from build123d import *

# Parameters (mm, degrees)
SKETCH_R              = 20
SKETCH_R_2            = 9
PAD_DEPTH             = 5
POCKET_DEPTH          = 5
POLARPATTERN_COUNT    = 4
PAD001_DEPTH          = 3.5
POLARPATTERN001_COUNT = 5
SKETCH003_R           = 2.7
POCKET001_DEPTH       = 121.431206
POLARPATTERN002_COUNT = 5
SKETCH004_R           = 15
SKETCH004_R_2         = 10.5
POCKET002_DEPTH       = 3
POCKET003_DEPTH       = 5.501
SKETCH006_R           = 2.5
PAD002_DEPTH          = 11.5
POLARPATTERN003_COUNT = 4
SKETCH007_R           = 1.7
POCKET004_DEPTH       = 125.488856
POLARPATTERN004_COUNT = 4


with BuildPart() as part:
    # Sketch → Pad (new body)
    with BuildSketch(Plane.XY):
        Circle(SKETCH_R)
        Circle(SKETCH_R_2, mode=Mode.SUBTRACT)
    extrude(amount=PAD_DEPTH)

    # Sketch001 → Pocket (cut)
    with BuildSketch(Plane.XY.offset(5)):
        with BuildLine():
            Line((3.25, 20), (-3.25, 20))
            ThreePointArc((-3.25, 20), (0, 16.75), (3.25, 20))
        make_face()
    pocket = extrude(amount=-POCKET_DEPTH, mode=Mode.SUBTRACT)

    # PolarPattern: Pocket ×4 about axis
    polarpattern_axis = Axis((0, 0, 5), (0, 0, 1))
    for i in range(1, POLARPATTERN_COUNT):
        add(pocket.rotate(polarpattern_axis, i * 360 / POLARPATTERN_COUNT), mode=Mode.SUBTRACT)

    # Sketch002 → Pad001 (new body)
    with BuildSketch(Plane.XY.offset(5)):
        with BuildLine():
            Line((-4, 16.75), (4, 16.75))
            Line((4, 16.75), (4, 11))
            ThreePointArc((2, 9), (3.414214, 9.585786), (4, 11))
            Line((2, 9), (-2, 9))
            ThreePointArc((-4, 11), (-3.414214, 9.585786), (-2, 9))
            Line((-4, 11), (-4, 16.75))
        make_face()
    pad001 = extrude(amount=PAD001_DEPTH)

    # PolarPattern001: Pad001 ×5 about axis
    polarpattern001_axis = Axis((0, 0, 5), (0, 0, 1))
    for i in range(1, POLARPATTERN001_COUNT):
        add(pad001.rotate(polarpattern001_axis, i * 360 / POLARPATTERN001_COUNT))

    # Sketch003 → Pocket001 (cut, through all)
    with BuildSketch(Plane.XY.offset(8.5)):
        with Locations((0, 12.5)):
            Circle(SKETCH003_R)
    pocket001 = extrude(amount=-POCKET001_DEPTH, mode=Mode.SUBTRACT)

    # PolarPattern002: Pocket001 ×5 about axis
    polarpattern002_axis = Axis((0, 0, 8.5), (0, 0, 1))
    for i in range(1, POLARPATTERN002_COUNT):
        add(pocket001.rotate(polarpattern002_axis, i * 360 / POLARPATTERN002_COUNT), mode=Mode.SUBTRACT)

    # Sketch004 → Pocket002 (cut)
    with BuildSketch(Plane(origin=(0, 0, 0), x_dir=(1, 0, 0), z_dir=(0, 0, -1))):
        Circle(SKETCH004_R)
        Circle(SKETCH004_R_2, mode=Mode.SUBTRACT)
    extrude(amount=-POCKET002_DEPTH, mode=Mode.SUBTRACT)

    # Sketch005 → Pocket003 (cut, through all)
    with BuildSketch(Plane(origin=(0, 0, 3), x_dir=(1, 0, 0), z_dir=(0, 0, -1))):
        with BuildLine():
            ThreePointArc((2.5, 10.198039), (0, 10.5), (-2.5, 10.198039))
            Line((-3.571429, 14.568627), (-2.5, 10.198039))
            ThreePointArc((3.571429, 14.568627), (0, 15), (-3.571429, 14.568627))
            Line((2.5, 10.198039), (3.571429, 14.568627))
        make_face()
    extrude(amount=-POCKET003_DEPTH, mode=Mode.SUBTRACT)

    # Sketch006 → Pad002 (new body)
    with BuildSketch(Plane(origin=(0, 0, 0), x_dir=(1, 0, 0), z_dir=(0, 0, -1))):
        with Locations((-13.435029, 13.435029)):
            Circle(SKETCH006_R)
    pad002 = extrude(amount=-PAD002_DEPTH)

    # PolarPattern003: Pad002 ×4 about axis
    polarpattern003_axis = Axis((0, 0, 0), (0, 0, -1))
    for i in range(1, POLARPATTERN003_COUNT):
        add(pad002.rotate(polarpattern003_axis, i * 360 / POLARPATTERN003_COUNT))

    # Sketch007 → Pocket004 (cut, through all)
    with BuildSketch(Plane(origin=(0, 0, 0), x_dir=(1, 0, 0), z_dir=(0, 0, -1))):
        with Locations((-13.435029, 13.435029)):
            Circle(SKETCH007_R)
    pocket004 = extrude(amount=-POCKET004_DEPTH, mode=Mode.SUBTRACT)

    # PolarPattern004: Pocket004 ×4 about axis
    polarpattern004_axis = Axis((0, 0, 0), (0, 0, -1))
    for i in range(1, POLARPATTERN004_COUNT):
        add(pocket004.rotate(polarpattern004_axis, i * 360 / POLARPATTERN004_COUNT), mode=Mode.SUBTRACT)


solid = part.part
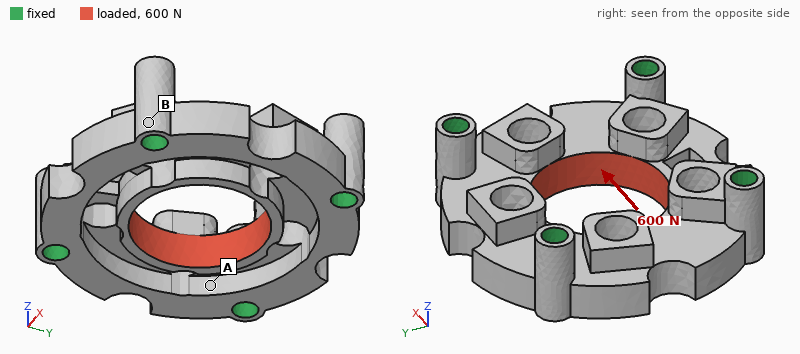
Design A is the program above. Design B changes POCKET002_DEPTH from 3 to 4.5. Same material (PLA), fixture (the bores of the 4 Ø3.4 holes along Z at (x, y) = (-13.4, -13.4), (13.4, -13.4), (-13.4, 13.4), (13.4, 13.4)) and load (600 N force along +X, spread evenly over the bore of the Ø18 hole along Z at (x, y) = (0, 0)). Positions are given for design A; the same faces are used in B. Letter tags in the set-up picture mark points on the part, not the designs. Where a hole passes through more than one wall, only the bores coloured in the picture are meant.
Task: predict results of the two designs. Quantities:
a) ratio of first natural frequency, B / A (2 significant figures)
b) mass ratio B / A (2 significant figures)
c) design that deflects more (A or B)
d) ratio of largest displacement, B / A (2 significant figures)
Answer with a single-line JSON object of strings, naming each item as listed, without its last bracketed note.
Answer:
{"ratio of first natural frequency, B / A": "0.71", "mass ratio B / A": "0.92", "design that deflects more": "B", "ratio of largest displacement, B / A": "2.2"}
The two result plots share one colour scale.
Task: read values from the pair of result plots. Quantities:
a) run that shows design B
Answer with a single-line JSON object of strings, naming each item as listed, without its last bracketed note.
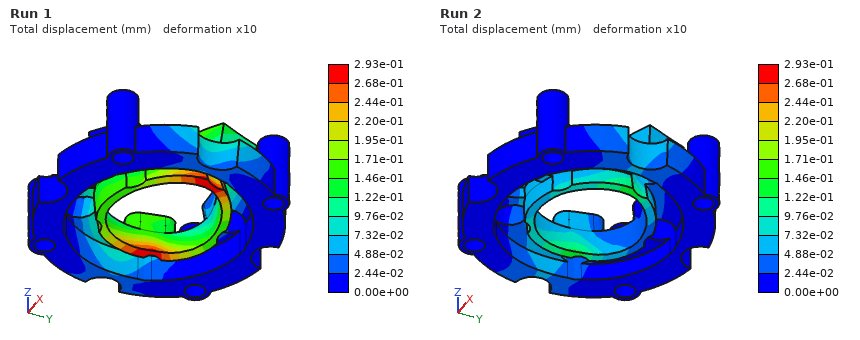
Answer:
{"run that shows design B": "Run 1"}
